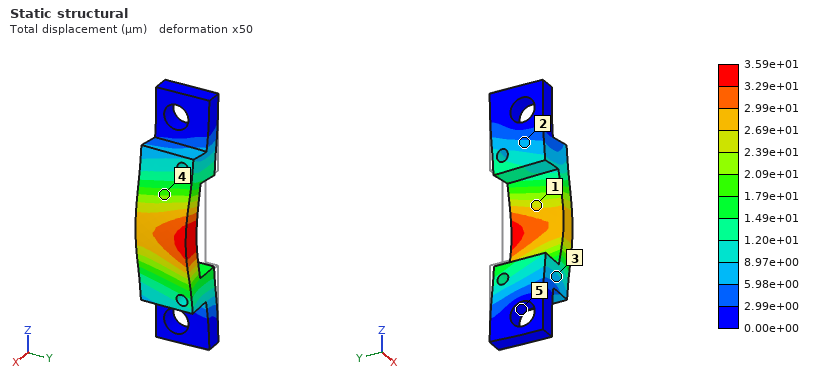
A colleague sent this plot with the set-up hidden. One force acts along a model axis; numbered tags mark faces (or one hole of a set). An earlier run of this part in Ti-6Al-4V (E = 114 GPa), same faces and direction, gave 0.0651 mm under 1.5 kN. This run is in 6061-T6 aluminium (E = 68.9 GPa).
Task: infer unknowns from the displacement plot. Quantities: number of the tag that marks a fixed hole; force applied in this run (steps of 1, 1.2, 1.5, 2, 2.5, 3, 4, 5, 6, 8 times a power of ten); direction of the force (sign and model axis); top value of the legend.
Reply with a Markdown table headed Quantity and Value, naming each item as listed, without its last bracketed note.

| Quantity | Value |
|---|---|
| number of the tag that marks a fixed hole | 5 |
| force applied in this run | 500 N |
| direction of the force | +X |
| top value of the legend | 3.59e+01 µm |
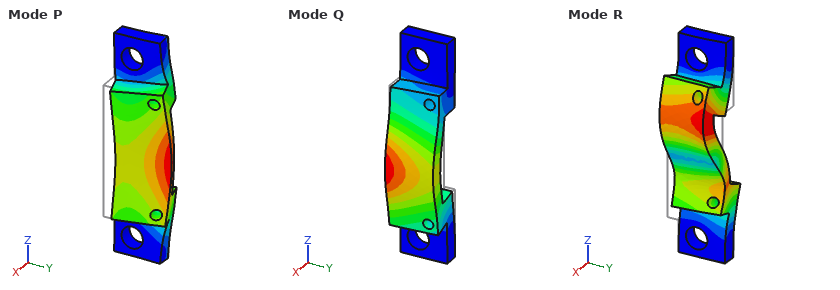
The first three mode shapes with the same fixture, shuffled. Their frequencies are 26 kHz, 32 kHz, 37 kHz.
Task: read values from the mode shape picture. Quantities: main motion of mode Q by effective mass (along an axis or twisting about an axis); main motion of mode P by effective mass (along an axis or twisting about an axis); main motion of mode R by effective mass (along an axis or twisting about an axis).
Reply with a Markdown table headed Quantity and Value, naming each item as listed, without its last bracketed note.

| Quantity | Value |
|---|---|
| main motion of mode Q by effective mass | along X |
| main motion of mode P by effective mass | along Y |
| main motion of mode R by effective mass | along Z |
